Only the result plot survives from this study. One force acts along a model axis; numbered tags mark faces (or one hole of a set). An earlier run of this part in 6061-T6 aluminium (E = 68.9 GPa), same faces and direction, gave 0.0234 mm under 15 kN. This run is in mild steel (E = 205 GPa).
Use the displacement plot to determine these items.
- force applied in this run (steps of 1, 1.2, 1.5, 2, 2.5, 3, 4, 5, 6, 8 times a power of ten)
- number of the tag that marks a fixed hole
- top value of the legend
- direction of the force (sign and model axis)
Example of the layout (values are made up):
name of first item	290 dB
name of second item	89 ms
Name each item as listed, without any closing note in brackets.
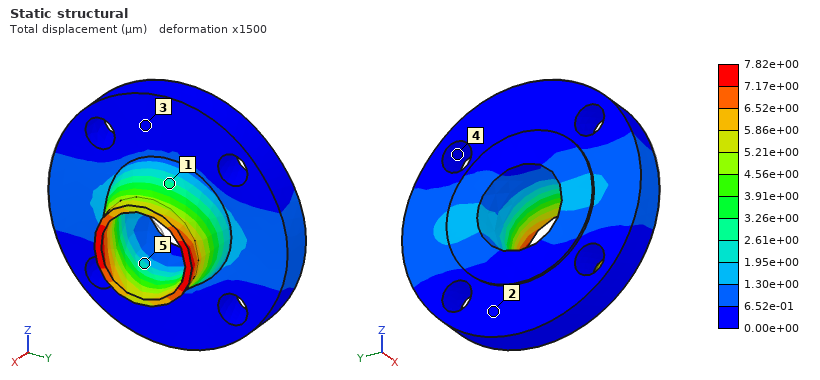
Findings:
force applied in this run	15 kN
number of the tag that marks a fixed hole	4
top value of the legend	7.82e+00 µm
direction of the force	+Y
